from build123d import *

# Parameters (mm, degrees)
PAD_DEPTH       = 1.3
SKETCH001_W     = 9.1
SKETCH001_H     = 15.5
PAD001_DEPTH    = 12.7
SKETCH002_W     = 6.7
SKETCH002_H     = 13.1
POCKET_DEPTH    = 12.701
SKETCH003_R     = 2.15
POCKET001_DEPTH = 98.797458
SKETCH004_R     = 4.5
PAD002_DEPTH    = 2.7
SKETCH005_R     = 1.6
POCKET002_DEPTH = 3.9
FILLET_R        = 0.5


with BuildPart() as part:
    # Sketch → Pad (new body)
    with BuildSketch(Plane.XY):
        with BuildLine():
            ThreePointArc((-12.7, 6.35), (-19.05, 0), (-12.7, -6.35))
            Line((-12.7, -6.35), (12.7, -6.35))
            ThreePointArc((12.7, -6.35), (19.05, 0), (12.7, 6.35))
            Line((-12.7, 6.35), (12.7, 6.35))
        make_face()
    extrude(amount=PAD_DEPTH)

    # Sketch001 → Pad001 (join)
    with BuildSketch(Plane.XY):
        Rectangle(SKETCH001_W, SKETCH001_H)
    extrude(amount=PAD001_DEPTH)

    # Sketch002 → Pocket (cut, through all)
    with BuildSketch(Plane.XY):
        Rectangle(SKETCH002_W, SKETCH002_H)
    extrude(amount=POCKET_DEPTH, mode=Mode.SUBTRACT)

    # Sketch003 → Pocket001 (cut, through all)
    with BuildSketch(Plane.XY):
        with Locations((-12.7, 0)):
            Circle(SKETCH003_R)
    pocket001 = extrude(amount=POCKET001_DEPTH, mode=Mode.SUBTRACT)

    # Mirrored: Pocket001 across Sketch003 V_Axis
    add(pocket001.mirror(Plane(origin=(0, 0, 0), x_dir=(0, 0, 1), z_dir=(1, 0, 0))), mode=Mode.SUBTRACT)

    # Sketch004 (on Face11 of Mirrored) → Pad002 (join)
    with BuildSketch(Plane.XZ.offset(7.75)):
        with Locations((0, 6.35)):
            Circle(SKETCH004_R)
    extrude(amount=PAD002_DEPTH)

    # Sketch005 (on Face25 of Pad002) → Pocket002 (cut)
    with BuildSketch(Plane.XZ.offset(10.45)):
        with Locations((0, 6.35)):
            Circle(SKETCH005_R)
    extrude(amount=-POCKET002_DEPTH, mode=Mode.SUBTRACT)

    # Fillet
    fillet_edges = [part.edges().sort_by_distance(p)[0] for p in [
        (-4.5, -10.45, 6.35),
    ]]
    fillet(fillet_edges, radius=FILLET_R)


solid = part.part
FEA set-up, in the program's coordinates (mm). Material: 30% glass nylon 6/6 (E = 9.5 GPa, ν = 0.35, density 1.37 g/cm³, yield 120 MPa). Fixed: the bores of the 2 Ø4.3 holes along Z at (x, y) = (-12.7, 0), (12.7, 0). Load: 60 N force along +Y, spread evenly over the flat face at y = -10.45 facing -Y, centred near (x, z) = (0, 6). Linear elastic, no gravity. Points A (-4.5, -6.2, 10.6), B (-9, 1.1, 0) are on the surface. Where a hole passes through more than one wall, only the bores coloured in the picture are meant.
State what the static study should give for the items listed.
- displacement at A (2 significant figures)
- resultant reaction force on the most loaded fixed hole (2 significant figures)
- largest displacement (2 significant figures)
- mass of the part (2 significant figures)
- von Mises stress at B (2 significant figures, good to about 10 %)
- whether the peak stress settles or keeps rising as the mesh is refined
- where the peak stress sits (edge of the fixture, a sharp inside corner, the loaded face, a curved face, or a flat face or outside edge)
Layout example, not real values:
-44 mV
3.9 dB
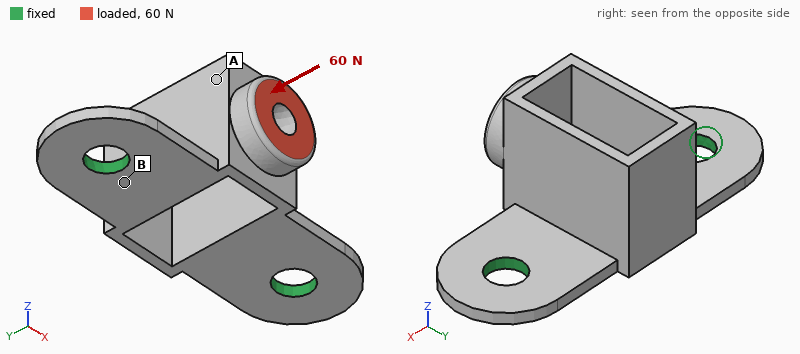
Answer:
0.28 mm
30 N
0.35 mm
1.7 g
25 MPa
keeps rising
edge of the fixture
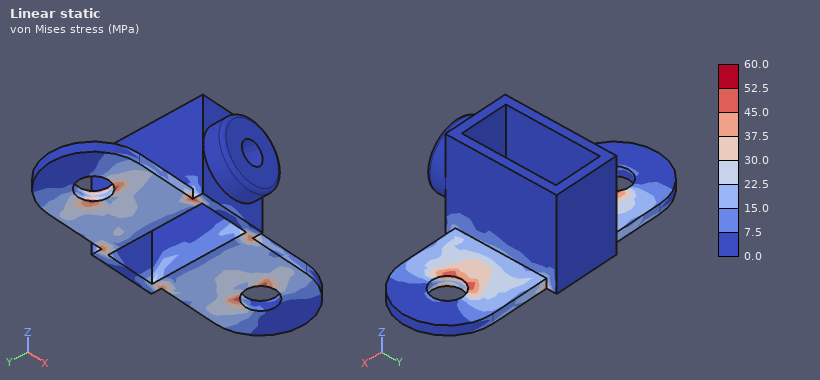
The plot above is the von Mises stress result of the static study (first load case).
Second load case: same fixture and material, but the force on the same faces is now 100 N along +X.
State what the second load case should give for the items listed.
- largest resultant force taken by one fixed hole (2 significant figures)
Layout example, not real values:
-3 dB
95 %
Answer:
83 N
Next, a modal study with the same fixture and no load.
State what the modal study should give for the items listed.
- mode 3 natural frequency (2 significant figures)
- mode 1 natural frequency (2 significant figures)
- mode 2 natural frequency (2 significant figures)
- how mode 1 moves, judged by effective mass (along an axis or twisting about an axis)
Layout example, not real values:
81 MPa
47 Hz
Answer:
4400 Hz
2000 Hz
4300 Hz
along Y
